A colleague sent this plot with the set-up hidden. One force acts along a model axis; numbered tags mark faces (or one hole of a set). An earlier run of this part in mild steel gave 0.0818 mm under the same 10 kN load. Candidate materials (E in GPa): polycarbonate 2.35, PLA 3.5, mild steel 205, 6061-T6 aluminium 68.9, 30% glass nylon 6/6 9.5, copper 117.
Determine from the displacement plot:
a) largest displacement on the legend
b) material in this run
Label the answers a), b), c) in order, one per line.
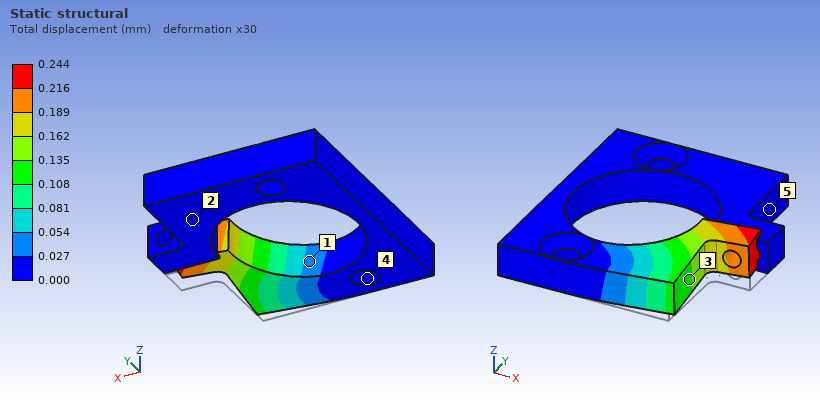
a) 0.244 mm
b) 6061-T6 aluminium
